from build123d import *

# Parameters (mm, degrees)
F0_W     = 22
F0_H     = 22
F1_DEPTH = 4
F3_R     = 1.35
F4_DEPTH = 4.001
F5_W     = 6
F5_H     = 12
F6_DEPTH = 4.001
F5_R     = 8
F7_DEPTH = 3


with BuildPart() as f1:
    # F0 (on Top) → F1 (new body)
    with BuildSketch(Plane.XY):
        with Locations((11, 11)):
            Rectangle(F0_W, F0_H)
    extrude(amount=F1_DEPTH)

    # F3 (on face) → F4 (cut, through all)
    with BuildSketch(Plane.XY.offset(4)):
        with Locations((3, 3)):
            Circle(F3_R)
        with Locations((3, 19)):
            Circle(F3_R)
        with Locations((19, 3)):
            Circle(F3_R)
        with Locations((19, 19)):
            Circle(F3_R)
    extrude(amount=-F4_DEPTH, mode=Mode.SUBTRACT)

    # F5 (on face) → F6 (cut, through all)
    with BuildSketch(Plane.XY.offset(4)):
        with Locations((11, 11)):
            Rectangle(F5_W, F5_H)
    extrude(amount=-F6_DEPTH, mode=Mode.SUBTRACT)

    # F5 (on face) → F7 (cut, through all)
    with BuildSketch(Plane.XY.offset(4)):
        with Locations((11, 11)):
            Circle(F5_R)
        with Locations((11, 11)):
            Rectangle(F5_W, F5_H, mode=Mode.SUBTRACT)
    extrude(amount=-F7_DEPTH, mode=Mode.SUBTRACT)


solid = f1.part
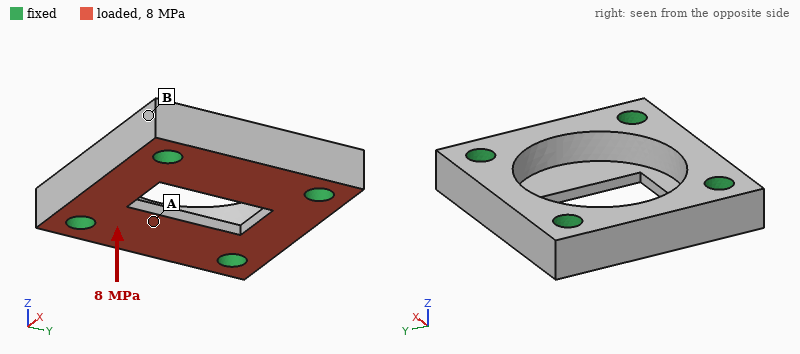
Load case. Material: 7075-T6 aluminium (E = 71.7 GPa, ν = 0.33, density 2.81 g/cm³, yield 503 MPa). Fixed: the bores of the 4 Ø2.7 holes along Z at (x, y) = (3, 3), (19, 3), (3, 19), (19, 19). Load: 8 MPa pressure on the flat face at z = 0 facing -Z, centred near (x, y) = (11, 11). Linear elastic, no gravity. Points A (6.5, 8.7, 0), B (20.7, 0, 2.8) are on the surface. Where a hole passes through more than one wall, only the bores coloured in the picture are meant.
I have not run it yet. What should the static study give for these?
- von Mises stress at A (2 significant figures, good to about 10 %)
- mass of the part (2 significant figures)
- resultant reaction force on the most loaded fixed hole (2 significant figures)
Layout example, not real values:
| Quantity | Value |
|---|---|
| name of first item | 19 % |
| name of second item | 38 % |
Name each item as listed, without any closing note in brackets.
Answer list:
| Quantity | Value |
|---|---|
| von Mises stress at A | 110 MPa |
| mass of the part | 3.3 g |
| resultant reaction force on the most loaded fixed hole | 780 N |
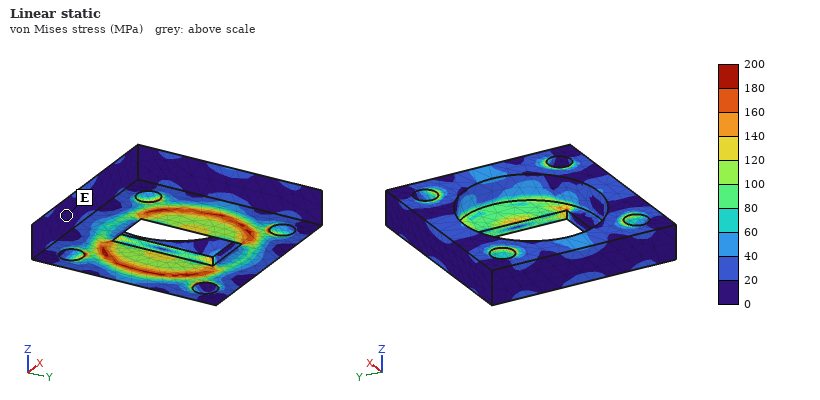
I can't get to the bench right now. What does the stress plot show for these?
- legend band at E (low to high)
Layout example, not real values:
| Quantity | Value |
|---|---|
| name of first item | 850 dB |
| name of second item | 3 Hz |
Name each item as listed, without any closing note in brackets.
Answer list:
| Quantity | Value |
|---|---|
| legend band at E | 0 to 20 MPa |
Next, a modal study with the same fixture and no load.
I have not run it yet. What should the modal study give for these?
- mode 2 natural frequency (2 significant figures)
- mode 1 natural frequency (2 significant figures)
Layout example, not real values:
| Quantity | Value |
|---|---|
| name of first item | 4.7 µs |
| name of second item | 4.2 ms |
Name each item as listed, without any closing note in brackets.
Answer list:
| Quantity | Value |
|---|---|
| mode 2 natural frequency | 46 kHz |
| mode 1 natural frequency | 46 kHz |
